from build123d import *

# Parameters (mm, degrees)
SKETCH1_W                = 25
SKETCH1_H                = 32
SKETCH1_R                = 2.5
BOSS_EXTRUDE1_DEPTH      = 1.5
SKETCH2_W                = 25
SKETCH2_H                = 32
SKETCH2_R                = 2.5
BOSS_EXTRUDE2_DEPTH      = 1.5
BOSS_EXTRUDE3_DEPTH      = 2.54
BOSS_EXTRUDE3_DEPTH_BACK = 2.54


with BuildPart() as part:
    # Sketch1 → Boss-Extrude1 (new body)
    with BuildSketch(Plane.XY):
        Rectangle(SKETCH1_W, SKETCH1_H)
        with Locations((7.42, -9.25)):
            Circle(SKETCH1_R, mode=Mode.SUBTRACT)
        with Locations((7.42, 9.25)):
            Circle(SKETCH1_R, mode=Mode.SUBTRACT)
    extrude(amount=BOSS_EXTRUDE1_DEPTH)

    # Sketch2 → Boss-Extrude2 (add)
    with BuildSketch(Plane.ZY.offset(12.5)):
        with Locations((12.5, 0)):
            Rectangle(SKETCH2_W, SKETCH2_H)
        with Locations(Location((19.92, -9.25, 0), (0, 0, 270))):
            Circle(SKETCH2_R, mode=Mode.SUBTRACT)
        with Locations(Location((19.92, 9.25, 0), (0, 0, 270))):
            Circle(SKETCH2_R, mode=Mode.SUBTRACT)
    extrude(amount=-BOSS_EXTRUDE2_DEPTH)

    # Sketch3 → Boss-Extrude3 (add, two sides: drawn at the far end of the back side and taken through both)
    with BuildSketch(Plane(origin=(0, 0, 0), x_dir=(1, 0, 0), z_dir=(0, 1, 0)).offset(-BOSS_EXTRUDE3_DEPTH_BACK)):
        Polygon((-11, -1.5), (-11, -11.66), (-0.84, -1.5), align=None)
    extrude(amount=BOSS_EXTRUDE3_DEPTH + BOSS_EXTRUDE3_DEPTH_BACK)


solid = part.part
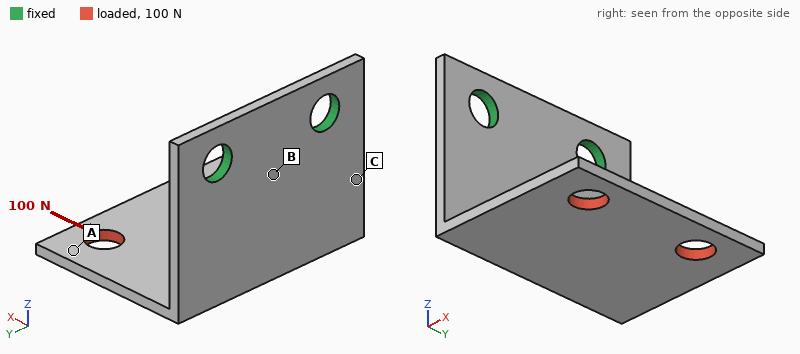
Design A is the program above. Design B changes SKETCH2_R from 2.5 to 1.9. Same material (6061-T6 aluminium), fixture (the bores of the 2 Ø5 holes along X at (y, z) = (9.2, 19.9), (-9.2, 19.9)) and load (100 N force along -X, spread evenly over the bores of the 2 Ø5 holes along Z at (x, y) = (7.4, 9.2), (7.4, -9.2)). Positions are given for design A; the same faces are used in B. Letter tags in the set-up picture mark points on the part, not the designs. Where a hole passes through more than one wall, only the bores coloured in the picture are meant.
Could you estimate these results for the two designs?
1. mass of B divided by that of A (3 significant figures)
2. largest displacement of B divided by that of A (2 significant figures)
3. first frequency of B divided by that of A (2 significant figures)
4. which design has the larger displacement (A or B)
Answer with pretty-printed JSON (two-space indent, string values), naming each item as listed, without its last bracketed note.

{
  "mass of B divided by that of A": "1.01",
  "largest displacement of B divided by that of A": "1.1",
  "first frequency of B divided by that of A": "0.95",
  "which design has the larger displacement": "B"
}
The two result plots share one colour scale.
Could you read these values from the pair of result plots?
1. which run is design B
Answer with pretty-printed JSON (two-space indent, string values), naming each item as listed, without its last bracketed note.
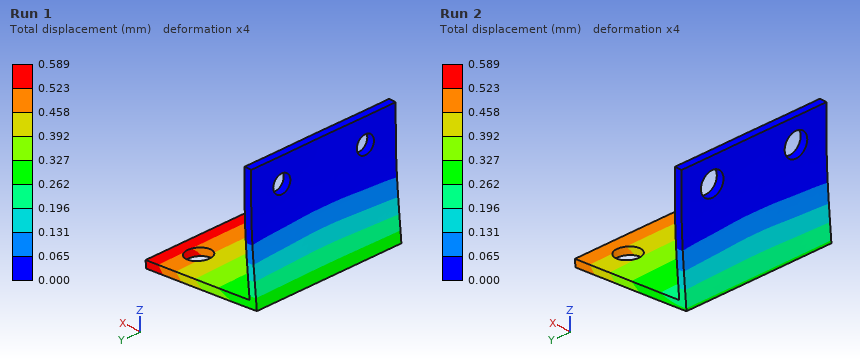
{
  "which run is design B": "Run 1"
}
